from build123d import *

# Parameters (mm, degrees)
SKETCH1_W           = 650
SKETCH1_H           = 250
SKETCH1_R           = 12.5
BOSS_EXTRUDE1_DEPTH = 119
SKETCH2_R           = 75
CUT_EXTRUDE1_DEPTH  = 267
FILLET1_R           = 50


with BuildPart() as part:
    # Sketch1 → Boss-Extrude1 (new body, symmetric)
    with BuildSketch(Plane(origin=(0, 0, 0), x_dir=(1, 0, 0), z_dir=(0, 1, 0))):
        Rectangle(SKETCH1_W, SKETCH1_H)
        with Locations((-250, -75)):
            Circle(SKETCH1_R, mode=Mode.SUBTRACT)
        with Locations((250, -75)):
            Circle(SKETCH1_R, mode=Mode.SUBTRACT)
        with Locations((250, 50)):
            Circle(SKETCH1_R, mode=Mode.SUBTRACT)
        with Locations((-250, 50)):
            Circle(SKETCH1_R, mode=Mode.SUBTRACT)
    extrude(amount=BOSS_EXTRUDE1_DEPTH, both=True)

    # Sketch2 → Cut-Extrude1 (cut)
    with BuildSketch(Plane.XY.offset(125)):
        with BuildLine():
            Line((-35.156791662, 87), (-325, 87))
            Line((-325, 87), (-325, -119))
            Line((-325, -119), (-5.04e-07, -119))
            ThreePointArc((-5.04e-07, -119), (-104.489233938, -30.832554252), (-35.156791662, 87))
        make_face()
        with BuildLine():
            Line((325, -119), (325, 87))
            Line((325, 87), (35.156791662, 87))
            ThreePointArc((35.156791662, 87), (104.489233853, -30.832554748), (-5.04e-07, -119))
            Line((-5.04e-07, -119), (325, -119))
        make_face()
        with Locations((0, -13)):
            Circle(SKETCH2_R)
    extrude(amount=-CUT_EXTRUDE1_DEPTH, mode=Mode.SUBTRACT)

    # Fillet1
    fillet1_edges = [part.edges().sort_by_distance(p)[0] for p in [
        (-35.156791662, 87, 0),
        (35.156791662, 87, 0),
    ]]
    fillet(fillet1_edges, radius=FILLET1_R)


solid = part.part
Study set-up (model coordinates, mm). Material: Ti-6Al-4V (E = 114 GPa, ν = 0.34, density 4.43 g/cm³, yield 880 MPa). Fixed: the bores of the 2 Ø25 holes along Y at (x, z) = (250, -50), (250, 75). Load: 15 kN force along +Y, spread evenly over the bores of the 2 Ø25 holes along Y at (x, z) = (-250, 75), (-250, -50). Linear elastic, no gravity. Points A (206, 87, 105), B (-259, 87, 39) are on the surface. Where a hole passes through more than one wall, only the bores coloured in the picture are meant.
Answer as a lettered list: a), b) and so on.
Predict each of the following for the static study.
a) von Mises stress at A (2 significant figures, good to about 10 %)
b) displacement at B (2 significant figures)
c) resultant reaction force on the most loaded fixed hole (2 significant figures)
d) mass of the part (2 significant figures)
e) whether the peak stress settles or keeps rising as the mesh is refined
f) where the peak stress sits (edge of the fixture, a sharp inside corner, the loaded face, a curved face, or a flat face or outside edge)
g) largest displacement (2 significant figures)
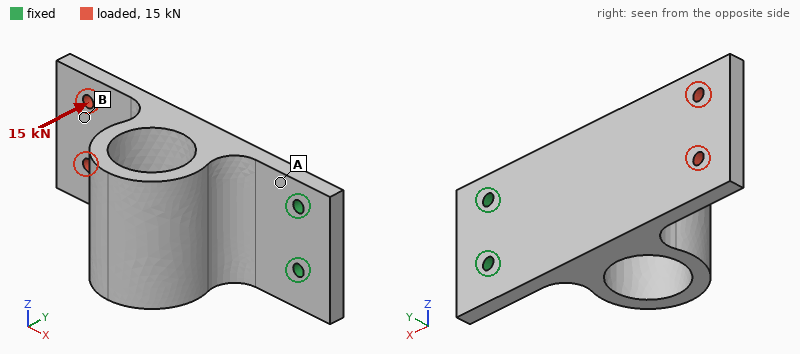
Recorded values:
a) 150 MPa
b) 5.3 mm
c) 7.7 kN
d) 46 kg
e) keeps rising
f) edge of the fixture
g) 6.2 mm
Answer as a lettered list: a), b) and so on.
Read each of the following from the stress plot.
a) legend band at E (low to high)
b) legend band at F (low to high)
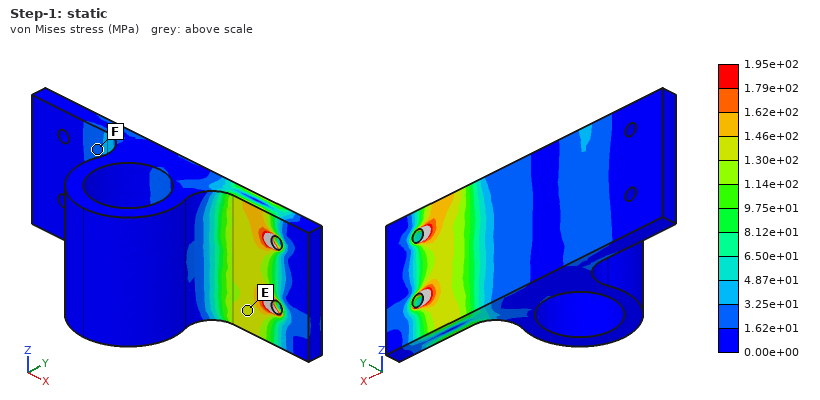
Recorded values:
a) 1.30e+02 to 1.46e+02 MPa
b) 1.62e+01 to 3.25e+01 MPa
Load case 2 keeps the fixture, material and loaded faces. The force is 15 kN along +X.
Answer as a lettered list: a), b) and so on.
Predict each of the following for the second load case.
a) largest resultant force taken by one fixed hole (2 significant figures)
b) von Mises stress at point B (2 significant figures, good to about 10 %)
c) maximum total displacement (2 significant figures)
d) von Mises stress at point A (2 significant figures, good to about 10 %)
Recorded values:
a) 7.6 kN
b) 1.1 MPa
c) 31 µm
d) 2.2 MPa
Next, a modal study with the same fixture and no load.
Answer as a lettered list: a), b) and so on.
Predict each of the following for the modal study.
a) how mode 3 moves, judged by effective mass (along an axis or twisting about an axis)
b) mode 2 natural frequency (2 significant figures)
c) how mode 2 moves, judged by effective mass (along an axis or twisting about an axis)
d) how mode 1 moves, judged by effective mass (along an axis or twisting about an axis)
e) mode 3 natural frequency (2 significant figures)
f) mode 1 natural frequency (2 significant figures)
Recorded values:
a) along Z
b) 280 Hz
c) along Z
d) along Y
e) 430 Hz
f) 72 Hz
